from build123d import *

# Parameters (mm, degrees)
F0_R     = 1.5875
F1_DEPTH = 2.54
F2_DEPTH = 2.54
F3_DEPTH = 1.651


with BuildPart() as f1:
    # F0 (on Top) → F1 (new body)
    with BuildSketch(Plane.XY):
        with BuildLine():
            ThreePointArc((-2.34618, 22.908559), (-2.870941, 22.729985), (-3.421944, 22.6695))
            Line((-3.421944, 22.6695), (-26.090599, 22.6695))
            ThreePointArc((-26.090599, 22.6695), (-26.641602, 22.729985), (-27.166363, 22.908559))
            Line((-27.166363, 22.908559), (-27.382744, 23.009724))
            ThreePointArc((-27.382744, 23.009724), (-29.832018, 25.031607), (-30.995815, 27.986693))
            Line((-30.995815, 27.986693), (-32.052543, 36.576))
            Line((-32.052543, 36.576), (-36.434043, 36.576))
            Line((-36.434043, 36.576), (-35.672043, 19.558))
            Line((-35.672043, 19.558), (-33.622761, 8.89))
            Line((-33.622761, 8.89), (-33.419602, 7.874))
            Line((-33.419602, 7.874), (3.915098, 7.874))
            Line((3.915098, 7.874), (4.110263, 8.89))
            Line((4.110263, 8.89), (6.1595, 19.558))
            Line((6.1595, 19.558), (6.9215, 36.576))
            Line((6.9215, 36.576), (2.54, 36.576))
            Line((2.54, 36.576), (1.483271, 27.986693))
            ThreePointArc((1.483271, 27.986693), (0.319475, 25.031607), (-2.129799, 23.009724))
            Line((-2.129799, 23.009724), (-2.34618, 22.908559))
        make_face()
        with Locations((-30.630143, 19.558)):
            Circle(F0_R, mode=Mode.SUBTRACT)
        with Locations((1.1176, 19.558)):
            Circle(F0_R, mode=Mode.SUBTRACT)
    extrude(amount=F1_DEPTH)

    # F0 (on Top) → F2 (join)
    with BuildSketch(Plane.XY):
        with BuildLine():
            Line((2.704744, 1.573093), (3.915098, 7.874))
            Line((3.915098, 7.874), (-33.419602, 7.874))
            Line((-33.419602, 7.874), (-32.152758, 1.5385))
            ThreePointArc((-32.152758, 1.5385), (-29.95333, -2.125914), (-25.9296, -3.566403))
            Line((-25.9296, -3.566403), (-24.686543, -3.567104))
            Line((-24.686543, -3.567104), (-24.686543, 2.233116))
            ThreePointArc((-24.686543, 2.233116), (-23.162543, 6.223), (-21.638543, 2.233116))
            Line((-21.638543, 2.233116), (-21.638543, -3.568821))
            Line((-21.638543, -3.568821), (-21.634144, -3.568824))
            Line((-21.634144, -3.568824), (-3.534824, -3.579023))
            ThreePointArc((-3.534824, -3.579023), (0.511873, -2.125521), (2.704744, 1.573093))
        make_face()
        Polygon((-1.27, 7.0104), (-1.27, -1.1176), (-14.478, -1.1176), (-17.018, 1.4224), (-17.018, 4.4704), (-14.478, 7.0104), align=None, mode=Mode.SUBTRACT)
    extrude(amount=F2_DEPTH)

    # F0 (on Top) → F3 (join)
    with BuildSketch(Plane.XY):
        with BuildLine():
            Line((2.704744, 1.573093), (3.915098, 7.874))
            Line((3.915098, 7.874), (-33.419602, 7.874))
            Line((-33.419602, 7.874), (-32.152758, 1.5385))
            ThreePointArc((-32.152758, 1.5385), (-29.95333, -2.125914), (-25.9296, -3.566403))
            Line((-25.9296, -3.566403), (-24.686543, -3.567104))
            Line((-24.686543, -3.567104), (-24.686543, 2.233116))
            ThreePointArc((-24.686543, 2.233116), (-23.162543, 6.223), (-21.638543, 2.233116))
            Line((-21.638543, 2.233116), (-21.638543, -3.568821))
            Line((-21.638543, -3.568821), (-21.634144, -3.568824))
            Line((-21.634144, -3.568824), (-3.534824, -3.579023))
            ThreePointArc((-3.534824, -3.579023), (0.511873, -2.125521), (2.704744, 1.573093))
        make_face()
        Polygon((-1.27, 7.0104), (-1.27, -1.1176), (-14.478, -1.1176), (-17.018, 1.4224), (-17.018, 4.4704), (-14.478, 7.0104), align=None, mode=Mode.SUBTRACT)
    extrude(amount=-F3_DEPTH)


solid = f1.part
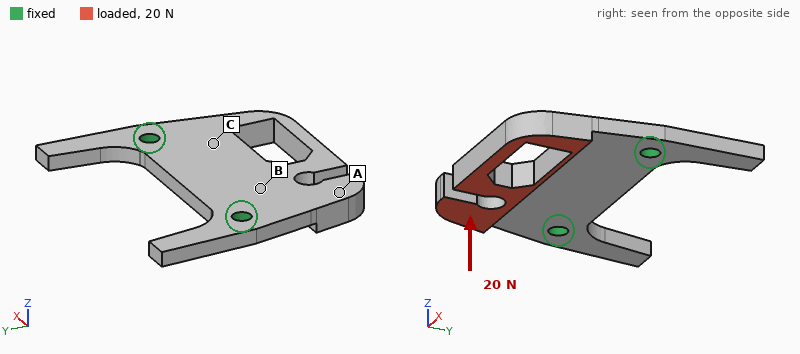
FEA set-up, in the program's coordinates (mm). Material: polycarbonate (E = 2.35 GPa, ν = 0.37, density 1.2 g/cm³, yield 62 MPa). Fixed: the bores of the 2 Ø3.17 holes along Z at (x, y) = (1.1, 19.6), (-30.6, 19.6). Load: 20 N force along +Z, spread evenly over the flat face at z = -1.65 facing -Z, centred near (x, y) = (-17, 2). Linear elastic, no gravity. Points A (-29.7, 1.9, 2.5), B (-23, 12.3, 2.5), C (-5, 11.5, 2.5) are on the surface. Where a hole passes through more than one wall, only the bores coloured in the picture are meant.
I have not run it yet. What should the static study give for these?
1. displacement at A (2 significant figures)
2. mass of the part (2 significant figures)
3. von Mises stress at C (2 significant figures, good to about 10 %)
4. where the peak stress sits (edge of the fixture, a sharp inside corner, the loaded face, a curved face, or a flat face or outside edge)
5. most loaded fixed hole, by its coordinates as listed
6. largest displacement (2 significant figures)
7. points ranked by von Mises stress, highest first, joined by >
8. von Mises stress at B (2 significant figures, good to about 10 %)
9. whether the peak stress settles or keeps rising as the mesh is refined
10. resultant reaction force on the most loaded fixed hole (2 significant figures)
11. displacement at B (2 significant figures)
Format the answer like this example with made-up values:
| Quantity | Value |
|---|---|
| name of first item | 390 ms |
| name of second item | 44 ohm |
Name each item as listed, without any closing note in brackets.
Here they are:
| Quantity | Value |
|---|---|
| displacement at A | 0.39 mm |
| mass of the part | 3.4 g |
| von Mises stress at C | 3.1 MPa |
| where the peak stress sits | edge of the fixture |
| most loaded fixed hole, by its coordinates as listed | (-30.6, 19.6) |
| largest displacement | 0.61 mm |
| points ranked by von Mises stress, highest first, joined by > | B > C > A |
| von Mises stress at B | 4.5 MPa |
| whether the peak stress settles or keeps rising as the mesh is refined | keeps rising |
| resultant reaction force on the most loaded fixed hole | 11 N |
| displacement at B | 0.13 mm |
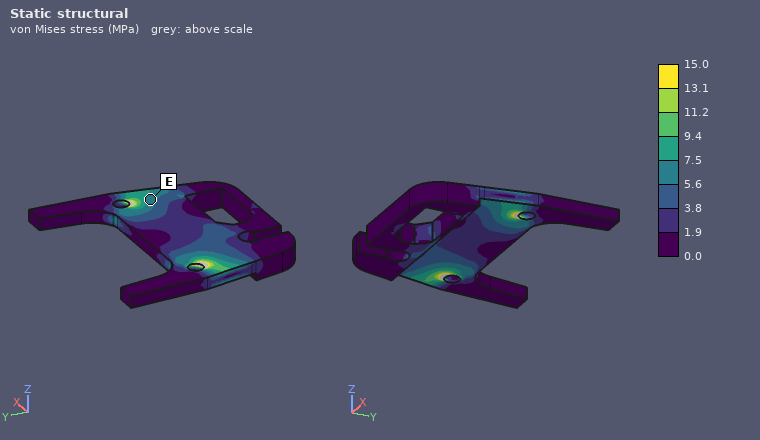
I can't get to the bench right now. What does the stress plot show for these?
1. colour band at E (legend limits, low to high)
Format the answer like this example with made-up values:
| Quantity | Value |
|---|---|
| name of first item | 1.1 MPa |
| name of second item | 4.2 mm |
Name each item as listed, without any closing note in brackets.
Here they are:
| Quantity | Value |
|---|---|
| colour band at E | 5.6 to 7.5 MPa |
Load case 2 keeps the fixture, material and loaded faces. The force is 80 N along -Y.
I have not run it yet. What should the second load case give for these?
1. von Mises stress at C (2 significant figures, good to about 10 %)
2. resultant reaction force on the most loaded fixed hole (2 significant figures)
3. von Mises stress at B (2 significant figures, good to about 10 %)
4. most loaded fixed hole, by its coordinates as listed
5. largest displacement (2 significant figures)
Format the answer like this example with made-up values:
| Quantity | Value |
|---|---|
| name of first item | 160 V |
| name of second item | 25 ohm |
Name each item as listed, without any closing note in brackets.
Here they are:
| Quantity | Value |
|---|---|
| von Mises stress at C | 3.4 MPa |
| resultant reaction force on the most loaded fixed hole | 47 N |
| von Mises stress at B | 4.7 MPa |
| most loaded fixed hole, by its coordinates as listed | (-30.6, 19.6) |
| largest displacement | 0.59 mm |
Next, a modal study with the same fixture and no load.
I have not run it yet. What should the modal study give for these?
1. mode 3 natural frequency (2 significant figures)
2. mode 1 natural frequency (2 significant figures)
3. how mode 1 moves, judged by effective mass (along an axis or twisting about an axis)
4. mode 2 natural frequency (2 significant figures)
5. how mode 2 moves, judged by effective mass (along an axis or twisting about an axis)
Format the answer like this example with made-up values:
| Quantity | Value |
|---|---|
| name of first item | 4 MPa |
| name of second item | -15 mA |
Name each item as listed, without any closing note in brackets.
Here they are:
| Quantity | Value |
|---|---|
| mode 3 natural frequency | 2500 Hz |
| mode 1 natural frequency | 950 Hz |
| how mode 1 moves, judged by effective mass | along Z |
| mode 2 natural frequency | 1900 Hz |
| how mode 2 moves, judged by effective mass | twisting about Y |
